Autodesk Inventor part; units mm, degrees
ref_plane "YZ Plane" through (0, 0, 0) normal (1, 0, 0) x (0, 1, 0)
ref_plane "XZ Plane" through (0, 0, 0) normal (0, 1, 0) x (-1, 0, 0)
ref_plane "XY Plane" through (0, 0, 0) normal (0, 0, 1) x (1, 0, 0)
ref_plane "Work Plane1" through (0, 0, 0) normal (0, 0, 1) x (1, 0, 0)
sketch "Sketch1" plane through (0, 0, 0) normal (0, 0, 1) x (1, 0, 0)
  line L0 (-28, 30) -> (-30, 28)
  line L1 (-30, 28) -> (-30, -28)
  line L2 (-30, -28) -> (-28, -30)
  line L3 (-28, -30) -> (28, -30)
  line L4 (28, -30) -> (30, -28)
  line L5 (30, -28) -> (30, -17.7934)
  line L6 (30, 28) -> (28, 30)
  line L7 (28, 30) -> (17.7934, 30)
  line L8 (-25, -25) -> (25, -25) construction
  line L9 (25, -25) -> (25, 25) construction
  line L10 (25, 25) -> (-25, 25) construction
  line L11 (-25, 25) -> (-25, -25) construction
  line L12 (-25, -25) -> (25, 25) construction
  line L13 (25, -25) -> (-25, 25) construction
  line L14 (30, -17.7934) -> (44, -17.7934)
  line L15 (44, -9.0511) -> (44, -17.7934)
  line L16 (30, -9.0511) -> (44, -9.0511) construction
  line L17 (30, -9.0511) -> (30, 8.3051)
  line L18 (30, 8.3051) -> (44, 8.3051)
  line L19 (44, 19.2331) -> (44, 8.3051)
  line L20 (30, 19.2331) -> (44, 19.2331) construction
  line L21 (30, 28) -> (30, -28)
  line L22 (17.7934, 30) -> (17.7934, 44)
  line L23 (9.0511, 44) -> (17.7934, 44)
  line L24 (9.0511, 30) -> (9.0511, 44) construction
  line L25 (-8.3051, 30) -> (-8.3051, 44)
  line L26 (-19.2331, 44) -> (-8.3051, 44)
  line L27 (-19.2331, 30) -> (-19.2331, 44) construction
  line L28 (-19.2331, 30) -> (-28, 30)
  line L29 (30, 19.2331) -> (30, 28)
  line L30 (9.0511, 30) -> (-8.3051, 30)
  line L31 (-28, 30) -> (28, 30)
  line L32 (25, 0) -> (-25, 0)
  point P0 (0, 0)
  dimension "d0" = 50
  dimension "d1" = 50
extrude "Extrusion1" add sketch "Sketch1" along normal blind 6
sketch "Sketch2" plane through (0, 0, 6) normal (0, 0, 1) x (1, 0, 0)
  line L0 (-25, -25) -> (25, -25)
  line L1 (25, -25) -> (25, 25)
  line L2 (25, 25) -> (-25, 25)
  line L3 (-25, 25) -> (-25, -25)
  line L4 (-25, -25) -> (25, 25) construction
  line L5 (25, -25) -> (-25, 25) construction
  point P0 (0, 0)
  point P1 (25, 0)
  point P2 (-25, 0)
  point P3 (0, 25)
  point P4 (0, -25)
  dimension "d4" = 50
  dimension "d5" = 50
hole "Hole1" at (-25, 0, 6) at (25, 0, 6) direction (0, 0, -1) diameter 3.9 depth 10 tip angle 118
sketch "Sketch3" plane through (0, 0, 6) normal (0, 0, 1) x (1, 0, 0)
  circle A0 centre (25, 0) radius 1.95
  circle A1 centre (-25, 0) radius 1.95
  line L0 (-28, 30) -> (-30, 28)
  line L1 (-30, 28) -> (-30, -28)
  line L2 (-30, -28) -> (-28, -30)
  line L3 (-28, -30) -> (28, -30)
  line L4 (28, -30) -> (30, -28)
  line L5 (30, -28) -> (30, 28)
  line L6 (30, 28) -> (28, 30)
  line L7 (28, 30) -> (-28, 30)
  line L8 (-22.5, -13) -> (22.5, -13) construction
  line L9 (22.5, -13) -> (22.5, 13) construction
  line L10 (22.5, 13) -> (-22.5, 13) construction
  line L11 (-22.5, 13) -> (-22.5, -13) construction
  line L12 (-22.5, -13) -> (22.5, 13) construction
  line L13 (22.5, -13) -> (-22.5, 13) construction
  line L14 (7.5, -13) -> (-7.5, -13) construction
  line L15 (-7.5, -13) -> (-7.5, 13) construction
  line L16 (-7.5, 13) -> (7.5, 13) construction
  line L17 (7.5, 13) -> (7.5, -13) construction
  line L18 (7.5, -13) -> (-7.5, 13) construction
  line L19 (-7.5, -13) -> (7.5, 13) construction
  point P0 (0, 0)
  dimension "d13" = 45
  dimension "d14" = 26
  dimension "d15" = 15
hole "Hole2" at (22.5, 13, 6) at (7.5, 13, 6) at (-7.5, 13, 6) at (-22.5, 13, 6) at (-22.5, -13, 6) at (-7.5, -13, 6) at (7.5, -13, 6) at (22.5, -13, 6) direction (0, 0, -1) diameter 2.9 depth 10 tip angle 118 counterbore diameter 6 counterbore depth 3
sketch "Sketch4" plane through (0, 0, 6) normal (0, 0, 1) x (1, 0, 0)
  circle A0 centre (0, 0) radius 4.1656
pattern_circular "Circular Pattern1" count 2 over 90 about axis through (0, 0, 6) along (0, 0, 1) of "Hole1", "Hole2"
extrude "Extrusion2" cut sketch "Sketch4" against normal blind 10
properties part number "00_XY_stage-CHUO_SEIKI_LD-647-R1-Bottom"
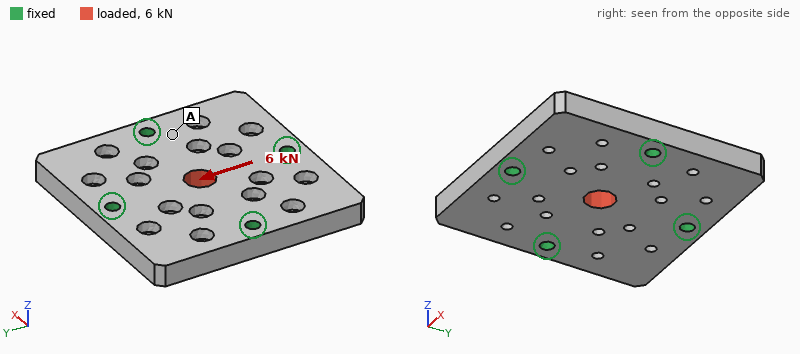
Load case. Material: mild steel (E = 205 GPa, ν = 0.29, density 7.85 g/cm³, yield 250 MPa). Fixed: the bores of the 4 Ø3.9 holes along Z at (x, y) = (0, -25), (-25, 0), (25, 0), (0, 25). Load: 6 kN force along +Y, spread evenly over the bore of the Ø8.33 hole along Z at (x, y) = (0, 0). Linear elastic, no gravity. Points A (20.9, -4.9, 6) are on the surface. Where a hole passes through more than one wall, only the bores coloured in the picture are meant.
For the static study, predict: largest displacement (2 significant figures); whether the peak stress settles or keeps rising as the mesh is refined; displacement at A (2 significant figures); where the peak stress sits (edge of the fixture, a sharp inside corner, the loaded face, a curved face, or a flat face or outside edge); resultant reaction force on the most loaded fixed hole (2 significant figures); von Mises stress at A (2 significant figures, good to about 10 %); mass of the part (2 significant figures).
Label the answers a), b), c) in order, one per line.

a) 3.4 µm
b) keeps rising
c) 0.57 µm
d) edge of the fixture
e) 2.0 kN
f) 9.7 MPa
g) 150 g
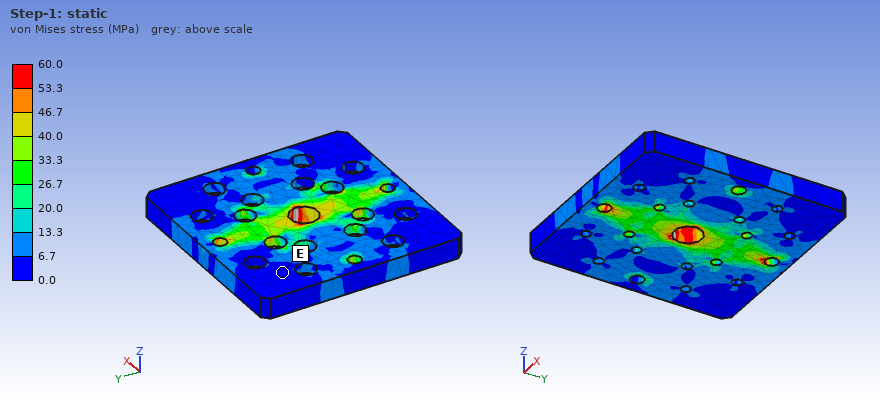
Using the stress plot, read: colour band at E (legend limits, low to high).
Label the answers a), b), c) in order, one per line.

a) 0.0 to 6.7 MPa
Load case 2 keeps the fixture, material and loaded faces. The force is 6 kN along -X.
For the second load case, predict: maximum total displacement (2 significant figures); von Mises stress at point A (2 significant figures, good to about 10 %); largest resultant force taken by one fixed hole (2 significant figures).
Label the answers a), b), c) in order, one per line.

a) 3.4 µm
b) 13 MPa
c) 2.0 kN
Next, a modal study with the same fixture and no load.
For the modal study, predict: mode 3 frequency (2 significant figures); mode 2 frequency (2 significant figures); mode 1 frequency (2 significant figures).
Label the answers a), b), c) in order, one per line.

a) 10 kHz
b) 10 kHz
c) 9700 Hz
